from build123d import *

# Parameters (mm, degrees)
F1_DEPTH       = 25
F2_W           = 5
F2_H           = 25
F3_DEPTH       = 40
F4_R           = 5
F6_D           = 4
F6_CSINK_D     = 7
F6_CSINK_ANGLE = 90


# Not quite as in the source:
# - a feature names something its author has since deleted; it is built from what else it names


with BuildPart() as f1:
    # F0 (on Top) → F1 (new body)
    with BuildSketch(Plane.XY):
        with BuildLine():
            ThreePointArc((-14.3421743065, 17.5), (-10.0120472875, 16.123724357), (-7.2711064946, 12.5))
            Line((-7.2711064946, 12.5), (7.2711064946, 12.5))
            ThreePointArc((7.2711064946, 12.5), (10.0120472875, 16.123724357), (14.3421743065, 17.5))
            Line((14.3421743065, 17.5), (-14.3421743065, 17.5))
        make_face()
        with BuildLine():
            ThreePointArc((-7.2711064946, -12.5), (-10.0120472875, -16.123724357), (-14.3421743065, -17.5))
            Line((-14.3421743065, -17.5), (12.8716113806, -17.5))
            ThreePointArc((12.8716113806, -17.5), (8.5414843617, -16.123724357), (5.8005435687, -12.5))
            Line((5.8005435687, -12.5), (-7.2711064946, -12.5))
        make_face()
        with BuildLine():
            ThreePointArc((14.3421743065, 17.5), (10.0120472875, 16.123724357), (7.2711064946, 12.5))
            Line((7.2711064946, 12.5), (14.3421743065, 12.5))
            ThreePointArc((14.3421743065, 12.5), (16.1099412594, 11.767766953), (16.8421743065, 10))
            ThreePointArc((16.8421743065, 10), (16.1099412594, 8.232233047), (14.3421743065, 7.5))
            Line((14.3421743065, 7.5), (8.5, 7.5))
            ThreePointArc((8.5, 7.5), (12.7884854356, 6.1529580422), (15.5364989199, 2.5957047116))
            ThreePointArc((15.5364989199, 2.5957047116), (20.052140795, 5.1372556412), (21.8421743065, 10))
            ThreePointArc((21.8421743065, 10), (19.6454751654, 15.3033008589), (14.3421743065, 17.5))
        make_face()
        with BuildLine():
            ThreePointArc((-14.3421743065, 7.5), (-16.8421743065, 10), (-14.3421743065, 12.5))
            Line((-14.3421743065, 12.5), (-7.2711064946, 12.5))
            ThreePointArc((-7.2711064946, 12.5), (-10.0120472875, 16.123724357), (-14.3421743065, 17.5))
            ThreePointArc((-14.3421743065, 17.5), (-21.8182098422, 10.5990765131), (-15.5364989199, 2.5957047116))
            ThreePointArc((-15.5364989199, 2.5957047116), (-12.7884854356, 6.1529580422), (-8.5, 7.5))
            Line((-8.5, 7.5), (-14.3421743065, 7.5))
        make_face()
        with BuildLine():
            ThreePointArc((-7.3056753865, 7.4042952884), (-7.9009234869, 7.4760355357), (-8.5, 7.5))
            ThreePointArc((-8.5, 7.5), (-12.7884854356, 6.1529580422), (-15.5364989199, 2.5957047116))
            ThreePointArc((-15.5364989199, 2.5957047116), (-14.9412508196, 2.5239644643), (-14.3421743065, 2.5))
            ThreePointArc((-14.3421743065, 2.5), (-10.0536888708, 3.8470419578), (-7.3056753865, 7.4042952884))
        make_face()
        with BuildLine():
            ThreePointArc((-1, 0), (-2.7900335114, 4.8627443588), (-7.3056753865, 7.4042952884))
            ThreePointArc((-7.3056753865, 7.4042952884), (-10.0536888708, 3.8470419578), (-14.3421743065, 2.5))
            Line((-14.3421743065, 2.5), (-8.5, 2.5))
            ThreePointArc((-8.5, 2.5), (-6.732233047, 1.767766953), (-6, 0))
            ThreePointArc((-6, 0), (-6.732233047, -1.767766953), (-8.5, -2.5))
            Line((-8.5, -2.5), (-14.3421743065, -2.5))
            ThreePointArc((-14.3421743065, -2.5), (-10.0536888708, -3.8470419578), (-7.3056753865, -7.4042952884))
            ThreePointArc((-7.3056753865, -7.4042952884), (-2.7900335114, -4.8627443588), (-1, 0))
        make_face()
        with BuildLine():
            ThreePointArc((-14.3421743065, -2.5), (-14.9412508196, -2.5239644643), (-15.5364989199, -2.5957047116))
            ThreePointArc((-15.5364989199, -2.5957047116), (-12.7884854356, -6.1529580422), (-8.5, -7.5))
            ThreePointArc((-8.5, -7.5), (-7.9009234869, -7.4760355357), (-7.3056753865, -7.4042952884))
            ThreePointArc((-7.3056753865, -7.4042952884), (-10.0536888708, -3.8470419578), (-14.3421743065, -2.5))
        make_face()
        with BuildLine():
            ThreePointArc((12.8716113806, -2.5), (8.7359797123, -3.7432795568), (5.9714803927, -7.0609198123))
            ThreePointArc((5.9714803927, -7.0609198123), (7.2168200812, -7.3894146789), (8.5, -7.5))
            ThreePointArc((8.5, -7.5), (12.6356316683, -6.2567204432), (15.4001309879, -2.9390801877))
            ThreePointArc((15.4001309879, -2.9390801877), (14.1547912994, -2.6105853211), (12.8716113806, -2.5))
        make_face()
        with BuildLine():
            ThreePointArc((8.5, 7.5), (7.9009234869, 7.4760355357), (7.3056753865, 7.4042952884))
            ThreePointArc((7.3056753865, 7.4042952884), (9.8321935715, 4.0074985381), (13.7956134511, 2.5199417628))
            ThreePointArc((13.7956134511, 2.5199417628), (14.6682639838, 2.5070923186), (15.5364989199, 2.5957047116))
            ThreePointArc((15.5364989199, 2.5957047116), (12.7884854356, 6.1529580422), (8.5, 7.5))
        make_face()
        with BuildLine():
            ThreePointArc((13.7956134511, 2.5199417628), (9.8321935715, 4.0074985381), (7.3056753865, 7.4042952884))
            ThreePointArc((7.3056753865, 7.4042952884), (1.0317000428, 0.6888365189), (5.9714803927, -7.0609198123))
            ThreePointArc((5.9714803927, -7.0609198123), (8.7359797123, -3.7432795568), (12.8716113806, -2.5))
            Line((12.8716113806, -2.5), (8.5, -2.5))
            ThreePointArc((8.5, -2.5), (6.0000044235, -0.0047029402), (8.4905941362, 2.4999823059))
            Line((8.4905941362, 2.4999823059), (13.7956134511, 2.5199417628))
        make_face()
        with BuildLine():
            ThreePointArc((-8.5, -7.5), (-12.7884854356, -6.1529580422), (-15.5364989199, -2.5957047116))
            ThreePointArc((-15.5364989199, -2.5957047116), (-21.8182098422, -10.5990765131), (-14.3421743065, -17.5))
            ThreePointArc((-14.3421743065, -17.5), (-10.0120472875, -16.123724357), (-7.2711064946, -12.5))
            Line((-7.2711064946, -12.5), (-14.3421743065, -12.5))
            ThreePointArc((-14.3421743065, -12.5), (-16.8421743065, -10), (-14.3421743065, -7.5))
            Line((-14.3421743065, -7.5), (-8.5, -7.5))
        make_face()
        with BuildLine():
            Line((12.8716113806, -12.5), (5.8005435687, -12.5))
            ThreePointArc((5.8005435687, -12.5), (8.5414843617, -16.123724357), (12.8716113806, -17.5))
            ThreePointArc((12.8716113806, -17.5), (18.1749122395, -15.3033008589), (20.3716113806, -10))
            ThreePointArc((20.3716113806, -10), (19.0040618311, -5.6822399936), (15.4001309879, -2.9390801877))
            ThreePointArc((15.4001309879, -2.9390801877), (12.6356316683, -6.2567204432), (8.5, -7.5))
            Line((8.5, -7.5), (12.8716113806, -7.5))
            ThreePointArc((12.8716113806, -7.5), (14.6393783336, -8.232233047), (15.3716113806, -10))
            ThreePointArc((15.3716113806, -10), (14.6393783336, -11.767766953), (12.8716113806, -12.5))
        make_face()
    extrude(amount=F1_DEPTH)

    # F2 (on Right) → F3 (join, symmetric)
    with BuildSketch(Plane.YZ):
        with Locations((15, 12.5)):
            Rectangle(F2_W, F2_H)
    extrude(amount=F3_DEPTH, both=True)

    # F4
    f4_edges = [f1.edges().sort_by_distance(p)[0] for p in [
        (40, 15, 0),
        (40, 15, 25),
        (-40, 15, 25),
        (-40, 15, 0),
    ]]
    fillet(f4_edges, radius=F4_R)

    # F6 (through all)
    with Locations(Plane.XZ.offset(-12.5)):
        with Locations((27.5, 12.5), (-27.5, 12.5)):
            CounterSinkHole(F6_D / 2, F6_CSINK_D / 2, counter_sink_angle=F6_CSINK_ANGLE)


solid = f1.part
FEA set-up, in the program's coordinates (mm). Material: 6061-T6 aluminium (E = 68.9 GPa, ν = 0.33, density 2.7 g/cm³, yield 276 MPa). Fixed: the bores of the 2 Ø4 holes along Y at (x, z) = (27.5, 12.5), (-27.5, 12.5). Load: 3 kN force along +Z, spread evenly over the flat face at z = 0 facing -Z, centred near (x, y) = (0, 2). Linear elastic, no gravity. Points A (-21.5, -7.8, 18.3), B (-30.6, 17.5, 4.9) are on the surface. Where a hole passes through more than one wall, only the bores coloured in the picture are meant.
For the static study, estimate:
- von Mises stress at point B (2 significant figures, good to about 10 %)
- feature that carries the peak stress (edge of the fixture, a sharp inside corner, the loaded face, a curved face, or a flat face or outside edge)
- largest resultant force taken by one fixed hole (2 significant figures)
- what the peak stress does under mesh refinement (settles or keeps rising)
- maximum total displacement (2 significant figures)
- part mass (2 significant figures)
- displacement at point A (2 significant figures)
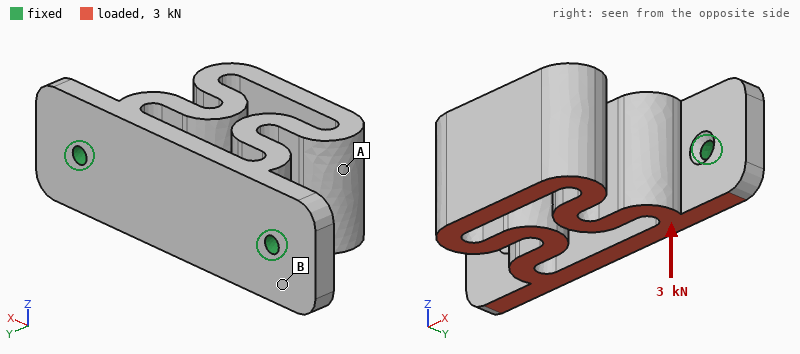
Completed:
62 MPa
edge of the fixture
1.5 kN
keeps rising
0.41 mm
71 g
0.27 mm
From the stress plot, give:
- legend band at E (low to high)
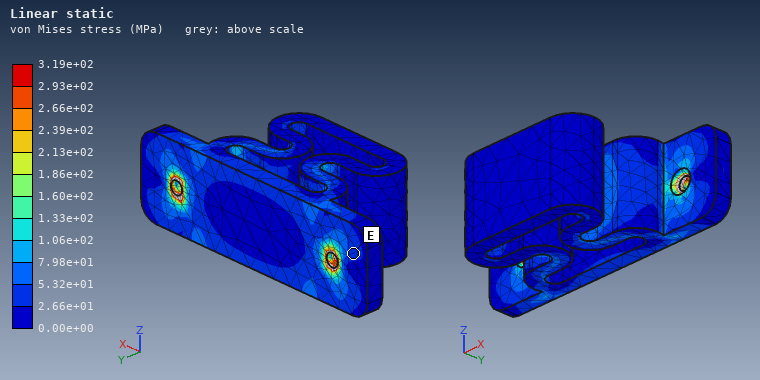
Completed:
2.66e+01 to 5.32e+01 MPa
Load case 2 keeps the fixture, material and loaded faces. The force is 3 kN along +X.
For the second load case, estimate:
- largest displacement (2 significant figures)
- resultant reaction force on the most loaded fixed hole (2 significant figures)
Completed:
0.23 mm
1.8 kN
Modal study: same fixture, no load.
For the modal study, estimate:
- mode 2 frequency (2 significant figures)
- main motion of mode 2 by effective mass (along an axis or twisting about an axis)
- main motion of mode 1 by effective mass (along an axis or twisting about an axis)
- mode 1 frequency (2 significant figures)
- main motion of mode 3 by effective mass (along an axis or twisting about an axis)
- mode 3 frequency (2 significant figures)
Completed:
2700 Hz
along X
along Z
1900 Hz
along Y
3400 Hz
